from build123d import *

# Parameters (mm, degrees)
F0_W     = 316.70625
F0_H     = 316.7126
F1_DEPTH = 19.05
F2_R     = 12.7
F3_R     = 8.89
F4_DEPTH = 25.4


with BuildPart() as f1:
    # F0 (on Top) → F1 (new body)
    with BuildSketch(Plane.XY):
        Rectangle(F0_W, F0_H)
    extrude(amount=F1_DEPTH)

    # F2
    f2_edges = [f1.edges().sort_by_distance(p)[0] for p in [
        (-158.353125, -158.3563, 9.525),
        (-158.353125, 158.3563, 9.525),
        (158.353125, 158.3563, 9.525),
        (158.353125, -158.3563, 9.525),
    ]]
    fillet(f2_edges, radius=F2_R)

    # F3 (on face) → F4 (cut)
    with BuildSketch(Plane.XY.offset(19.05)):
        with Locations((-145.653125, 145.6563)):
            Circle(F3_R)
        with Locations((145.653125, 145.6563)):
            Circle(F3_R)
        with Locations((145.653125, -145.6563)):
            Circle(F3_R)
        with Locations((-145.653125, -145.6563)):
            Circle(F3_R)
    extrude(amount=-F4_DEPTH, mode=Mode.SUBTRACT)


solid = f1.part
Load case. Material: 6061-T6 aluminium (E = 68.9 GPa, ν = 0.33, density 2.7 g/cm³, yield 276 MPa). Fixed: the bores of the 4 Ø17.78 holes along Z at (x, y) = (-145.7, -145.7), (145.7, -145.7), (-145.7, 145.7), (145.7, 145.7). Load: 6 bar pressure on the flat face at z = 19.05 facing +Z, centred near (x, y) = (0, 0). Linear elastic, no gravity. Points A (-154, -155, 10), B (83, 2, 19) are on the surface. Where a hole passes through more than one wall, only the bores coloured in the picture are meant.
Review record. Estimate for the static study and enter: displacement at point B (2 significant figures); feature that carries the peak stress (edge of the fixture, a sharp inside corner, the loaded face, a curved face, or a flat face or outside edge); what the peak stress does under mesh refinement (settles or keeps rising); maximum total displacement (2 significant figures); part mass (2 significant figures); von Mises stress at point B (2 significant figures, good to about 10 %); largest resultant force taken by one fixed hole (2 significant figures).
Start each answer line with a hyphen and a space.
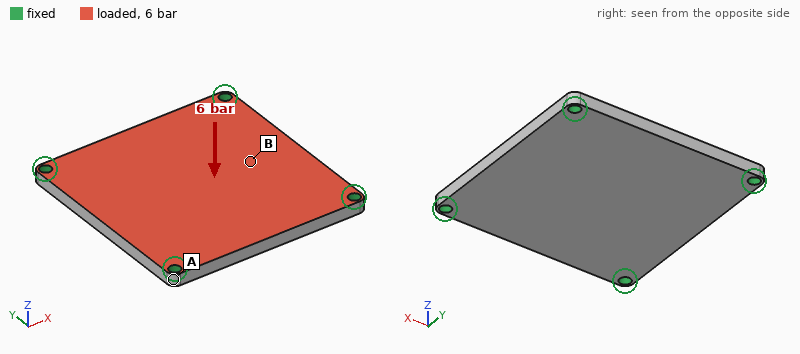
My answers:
- 0.70 mm
- edge of the fixture
- keeps rising
- 0.86 mm
- 5.1 kg
- 46 MPa
- 15 kN
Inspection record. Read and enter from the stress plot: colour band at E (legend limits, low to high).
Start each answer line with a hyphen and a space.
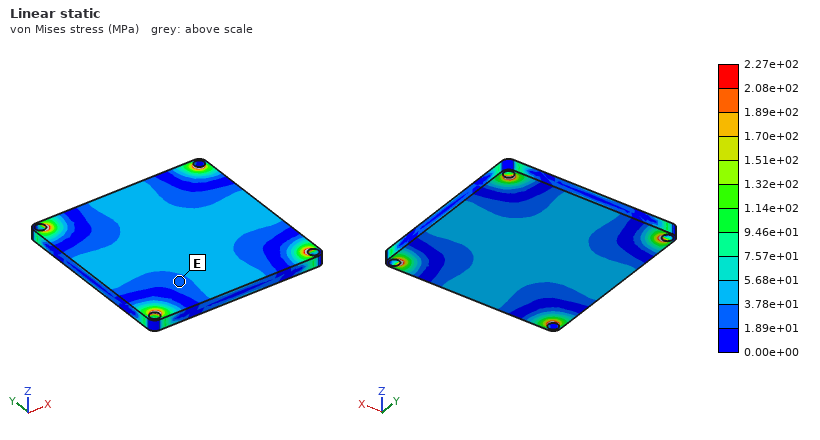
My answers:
- 1.89e+01 to 3.78e+01 MPa
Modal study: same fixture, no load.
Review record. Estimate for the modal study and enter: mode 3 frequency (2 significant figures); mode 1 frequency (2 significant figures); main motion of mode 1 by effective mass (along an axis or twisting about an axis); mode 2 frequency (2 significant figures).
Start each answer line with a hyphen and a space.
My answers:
- 1300 Hz
- 700 Hz
- along Z
- 1300 Hz
